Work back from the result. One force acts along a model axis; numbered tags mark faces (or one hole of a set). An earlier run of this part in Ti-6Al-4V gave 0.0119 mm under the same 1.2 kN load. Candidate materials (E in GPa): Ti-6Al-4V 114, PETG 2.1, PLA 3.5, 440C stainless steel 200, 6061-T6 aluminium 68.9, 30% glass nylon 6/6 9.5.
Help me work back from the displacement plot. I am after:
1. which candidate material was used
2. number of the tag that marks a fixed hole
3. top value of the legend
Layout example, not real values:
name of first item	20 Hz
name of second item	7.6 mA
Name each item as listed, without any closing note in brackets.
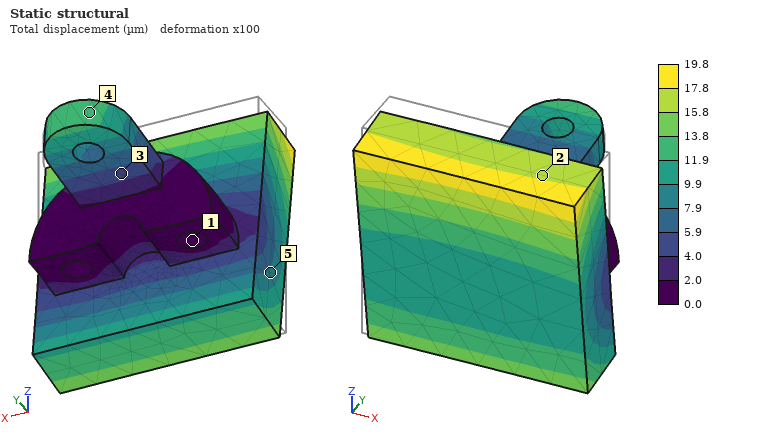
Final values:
which candidate material was used	6061-T6 aluminium
number of the tag that marks a fixed hole	1
top value of the legend	19.8 µm
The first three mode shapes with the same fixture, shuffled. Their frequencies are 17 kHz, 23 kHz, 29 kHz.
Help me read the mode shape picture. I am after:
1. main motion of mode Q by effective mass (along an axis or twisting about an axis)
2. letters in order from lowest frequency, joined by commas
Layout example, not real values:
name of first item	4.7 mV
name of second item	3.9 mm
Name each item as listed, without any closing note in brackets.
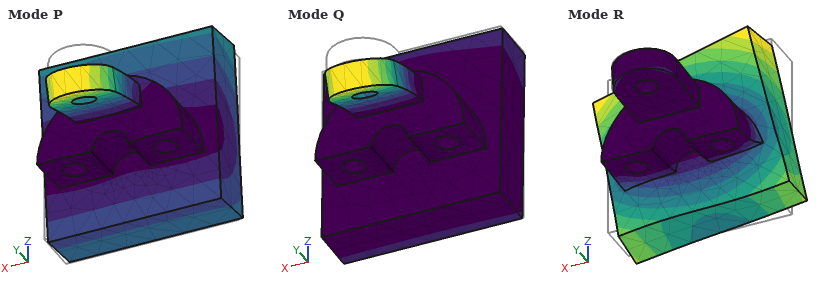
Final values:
main motion of mode Q by effective mass	along Z
letters in order from lowest frequency, joined by commas	P, Q, R
